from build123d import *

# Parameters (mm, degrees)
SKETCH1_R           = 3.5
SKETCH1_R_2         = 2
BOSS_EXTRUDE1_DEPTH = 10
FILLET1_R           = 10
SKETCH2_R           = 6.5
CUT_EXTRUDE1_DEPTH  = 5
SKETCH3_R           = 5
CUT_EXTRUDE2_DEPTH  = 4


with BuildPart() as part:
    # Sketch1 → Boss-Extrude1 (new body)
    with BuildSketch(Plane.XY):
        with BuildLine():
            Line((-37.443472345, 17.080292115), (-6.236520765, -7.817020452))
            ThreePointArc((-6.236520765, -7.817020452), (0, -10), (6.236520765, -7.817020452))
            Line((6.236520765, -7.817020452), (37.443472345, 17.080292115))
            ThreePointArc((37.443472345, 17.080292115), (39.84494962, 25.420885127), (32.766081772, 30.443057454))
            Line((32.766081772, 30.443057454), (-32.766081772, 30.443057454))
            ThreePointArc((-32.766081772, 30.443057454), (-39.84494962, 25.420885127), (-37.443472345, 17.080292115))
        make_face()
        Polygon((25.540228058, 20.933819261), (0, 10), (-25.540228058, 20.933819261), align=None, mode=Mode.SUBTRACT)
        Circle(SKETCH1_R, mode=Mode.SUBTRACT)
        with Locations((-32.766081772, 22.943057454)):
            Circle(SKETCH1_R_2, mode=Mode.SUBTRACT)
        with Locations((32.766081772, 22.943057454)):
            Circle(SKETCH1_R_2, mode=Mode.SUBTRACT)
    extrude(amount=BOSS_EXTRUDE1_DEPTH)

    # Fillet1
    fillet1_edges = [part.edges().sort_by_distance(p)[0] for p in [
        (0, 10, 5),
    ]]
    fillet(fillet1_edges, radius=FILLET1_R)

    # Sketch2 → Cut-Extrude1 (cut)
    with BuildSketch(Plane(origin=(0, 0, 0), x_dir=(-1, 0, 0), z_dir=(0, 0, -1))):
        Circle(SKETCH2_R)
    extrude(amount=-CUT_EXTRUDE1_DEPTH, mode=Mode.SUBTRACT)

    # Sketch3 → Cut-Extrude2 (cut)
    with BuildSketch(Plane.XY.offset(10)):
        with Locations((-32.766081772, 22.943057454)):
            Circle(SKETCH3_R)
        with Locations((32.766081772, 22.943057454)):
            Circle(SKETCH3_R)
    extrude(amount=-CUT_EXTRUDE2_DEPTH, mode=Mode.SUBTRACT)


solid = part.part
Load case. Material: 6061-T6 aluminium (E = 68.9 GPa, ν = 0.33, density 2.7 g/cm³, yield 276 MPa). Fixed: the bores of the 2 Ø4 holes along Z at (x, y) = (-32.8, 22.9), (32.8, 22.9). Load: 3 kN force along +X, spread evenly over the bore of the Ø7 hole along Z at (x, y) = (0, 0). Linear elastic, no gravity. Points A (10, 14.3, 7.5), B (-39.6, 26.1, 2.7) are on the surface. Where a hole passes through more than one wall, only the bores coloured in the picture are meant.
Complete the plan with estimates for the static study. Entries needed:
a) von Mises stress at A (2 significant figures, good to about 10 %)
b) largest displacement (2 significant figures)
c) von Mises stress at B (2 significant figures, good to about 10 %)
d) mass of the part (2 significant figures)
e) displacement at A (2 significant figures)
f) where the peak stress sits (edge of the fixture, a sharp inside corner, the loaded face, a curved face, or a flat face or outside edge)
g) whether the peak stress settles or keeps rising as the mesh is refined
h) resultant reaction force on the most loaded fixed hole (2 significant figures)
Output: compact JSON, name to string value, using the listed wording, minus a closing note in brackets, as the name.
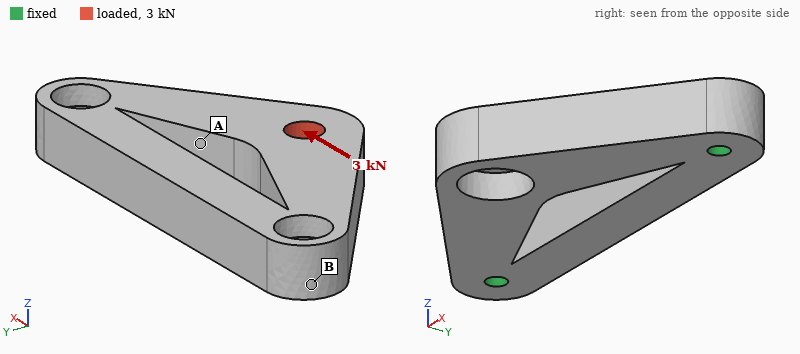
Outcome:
{"von Mises stress at A": "20 MPa", "largest displacement": "17 µm", "von Mises stress at B": "7.7 MPa", "mass of the part": "46 g", "displacement at A": "8.8 µm", "where the peak stress sits": "edge of the fixture", "whether the peak stress settles or keeps rising as the mesh is refined": "keeps rising", "resultant reaction force on the most loaded fixed hole": "1.8 kN"}
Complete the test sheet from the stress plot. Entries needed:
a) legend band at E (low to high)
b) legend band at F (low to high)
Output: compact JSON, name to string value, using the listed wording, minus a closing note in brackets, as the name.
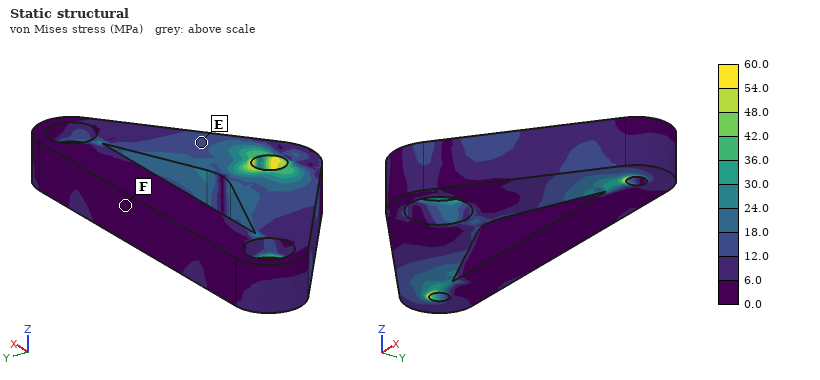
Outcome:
{"legend band at E": "12.0 to 18.0 MPa", "legend band at F": "0.0 to 6.0 MPa"}
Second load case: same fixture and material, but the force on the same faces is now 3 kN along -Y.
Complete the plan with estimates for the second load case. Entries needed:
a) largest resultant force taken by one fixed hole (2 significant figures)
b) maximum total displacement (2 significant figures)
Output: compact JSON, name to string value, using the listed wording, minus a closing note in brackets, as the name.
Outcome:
{"largest resultant force taken by one fixed hole": "2.0 kN", "maximum total displacement": "0.11 mm"}
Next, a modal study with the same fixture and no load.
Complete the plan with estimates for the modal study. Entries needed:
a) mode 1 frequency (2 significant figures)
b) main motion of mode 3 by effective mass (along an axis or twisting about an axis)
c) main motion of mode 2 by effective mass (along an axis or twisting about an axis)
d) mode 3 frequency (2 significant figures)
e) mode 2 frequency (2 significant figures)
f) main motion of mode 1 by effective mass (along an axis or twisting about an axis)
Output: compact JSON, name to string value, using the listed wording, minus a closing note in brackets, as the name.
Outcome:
{"mode 1 frequency": "4000 Hz", "main motion of mode 3 by effective mass": "along Y", "main motion of mode 2 by effective mass": "along Z", "mode 3 frequency": "10 kHz", "mode 2 frequency": "9000 Hz", "main motion of mode 1 by effective mass": "along Z"}
